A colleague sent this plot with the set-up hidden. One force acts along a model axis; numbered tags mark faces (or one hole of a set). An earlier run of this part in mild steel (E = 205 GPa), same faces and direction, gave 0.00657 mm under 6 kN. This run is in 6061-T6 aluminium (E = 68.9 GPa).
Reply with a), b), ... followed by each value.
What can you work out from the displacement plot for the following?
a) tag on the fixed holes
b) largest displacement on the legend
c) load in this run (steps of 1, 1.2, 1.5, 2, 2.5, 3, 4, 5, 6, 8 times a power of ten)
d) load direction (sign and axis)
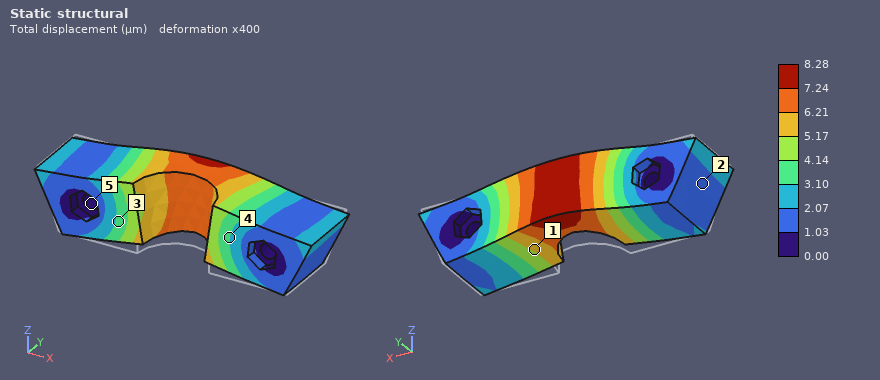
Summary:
a) 5
b) 8.28 µm
c) 2.5 kN
d) +Z
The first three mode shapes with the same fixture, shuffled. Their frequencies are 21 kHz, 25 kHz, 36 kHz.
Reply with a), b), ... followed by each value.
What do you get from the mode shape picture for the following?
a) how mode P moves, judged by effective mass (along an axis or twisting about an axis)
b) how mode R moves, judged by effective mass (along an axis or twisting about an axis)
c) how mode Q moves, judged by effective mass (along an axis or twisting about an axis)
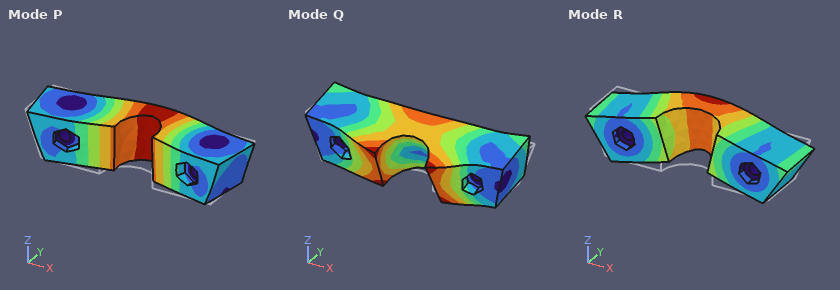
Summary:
a) along Y
b) along Z
c) twisting about X
